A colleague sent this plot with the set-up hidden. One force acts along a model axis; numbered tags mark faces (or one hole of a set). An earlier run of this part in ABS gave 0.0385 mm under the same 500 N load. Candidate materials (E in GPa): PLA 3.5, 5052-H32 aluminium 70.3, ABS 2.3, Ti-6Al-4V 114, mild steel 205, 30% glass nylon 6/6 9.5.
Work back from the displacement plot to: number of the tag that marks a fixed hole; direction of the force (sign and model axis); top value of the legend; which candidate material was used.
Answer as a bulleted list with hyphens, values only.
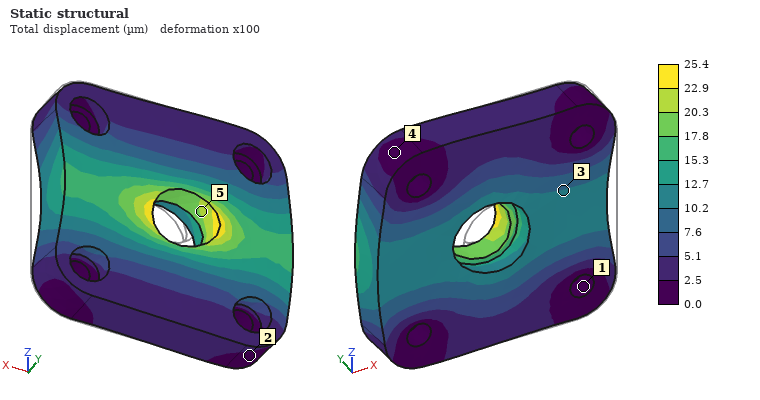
- 1
- -X
- 25.4 µm
- PLA
